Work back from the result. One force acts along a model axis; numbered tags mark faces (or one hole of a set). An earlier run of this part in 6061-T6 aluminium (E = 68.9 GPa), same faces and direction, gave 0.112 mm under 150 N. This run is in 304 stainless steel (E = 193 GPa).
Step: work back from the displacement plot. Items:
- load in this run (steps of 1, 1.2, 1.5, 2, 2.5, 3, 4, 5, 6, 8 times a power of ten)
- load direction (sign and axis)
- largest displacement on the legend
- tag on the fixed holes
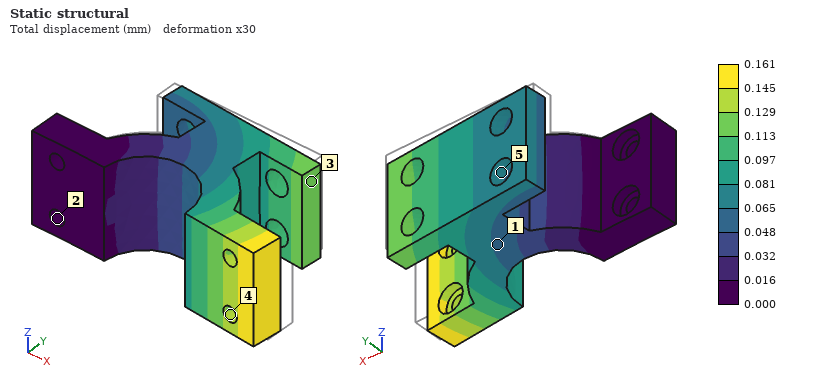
600 N
-Y
0.161 mm
2
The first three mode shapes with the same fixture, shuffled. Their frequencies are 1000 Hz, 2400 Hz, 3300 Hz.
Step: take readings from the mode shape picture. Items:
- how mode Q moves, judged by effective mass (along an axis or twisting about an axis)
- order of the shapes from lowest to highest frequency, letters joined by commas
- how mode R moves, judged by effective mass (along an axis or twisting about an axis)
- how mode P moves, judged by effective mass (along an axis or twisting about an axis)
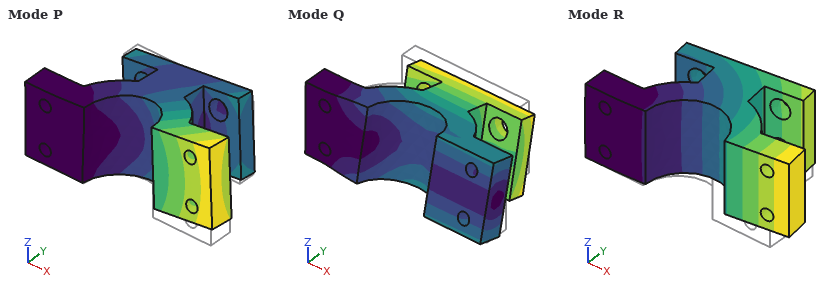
along Z
R, P, Q
along Y
along Z
